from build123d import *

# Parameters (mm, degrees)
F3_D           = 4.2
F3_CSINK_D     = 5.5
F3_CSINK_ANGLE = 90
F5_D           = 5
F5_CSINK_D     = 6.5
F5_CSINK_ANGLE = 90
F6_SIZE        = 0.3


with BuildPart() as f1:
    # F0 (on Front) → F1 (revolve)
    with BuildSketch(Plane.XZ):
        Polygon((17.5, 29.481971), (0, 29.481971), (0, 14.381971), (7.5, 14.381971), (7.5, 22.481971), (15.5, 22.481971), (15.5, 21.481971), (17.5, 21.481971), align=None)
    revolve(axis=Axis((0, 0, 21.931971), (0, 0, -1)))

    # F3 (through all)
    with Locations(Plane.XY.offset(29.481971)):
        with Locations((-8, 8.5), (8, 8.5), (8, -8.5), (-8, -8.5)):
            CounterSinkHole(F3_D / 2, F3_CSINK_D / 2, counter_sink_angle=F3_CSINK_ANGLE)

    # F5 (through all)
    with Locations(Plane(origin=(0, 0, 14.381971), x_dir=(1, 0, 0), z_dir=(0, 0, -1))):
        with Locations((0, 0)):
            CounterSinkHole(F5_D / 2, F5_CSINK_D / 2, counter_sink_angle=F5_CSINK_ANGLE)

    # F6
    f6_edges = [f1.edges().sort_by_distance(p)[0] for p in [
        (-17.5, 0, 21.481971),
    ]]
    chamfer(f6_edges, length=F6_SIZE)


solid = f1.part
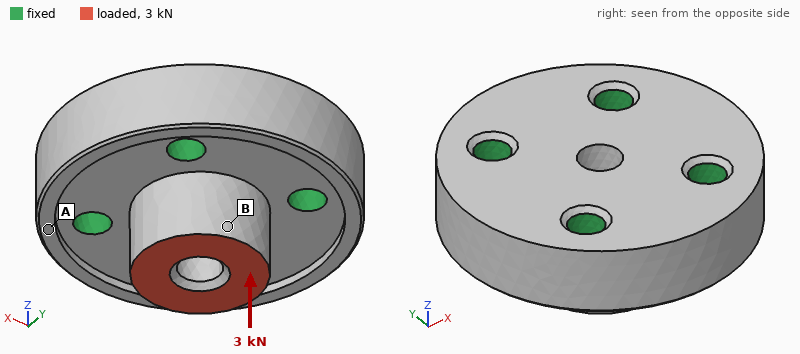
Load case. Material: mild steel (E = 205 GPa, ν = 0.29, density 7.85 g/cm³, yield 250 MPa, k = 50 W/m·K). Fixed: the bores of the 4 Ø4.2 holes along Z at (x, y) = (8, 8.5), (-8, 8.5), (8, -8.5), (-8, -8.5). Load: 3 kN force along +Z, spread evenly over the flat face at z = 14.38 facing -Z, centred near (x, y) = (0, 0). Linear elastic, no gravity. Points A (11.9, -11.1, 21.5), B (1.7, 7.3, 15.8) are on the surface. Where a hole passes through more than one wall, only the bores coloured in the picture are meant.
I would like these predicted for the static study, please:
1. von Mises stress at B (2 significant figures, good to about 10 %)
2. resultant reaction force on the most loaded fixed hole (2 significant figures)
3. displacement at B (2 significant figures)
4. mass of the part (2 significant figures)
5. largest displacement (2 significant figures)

21 MPa
770 N
1.7 µm
60 g
1.8 µm
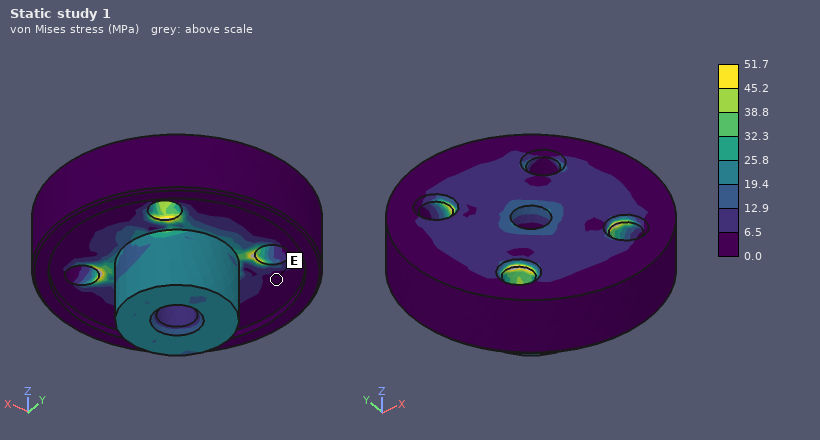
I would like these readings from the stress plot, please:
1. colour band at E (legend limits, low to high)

0.0 to 6.5 MPa
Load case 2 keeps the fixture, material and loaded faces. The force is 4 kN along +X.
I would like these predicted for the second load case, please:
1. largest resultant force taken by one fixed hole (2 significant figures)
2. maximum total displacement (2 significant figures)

1.8 kN
11 µm
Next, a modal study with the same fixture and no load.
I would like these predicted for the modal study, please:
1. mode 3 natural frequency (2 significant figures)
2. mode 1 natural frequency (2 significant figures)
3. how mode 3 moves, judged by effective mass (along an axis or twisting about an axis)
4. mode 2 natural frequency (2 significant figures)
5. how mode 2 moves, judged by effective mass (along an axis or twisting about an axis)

52 kHz
47 kHz
along Z
49 kHz
along Y
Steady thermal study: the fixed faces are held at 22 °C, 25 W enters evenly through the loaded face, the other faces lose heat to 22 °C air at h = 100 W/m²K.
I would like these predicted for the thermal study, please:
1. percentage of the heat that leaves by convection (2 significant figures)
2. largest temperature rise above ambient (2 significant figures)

7.3 %
37 K
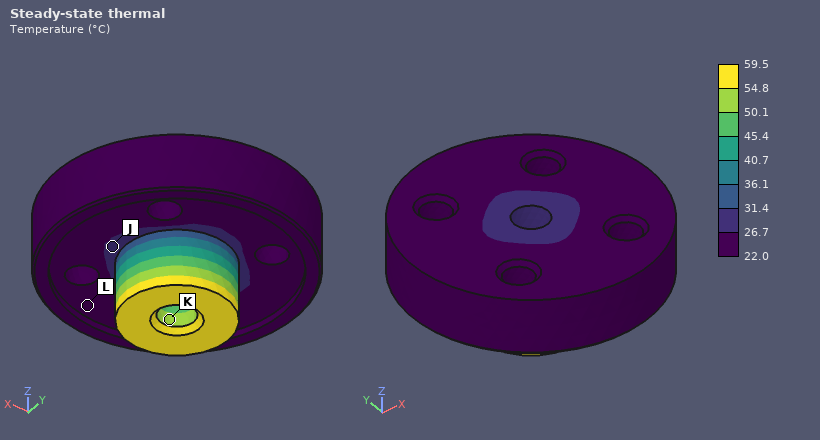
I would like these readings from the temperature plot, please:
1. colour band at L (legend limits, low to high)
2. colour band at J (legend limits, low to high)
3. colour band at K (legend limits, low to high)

22.0 to 26.7 °C
26.7 to 31.4 °C
50.1 to 54.8 °C
